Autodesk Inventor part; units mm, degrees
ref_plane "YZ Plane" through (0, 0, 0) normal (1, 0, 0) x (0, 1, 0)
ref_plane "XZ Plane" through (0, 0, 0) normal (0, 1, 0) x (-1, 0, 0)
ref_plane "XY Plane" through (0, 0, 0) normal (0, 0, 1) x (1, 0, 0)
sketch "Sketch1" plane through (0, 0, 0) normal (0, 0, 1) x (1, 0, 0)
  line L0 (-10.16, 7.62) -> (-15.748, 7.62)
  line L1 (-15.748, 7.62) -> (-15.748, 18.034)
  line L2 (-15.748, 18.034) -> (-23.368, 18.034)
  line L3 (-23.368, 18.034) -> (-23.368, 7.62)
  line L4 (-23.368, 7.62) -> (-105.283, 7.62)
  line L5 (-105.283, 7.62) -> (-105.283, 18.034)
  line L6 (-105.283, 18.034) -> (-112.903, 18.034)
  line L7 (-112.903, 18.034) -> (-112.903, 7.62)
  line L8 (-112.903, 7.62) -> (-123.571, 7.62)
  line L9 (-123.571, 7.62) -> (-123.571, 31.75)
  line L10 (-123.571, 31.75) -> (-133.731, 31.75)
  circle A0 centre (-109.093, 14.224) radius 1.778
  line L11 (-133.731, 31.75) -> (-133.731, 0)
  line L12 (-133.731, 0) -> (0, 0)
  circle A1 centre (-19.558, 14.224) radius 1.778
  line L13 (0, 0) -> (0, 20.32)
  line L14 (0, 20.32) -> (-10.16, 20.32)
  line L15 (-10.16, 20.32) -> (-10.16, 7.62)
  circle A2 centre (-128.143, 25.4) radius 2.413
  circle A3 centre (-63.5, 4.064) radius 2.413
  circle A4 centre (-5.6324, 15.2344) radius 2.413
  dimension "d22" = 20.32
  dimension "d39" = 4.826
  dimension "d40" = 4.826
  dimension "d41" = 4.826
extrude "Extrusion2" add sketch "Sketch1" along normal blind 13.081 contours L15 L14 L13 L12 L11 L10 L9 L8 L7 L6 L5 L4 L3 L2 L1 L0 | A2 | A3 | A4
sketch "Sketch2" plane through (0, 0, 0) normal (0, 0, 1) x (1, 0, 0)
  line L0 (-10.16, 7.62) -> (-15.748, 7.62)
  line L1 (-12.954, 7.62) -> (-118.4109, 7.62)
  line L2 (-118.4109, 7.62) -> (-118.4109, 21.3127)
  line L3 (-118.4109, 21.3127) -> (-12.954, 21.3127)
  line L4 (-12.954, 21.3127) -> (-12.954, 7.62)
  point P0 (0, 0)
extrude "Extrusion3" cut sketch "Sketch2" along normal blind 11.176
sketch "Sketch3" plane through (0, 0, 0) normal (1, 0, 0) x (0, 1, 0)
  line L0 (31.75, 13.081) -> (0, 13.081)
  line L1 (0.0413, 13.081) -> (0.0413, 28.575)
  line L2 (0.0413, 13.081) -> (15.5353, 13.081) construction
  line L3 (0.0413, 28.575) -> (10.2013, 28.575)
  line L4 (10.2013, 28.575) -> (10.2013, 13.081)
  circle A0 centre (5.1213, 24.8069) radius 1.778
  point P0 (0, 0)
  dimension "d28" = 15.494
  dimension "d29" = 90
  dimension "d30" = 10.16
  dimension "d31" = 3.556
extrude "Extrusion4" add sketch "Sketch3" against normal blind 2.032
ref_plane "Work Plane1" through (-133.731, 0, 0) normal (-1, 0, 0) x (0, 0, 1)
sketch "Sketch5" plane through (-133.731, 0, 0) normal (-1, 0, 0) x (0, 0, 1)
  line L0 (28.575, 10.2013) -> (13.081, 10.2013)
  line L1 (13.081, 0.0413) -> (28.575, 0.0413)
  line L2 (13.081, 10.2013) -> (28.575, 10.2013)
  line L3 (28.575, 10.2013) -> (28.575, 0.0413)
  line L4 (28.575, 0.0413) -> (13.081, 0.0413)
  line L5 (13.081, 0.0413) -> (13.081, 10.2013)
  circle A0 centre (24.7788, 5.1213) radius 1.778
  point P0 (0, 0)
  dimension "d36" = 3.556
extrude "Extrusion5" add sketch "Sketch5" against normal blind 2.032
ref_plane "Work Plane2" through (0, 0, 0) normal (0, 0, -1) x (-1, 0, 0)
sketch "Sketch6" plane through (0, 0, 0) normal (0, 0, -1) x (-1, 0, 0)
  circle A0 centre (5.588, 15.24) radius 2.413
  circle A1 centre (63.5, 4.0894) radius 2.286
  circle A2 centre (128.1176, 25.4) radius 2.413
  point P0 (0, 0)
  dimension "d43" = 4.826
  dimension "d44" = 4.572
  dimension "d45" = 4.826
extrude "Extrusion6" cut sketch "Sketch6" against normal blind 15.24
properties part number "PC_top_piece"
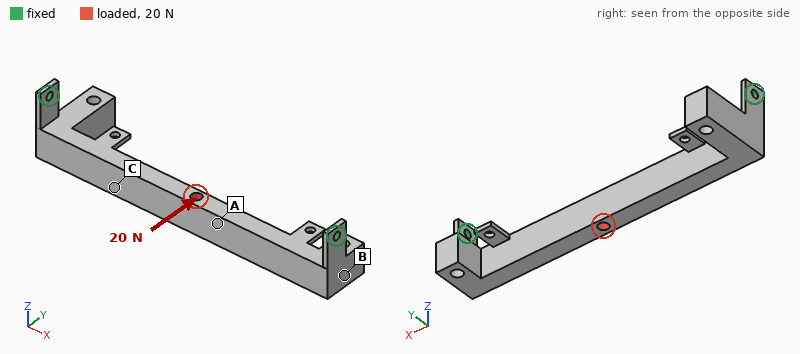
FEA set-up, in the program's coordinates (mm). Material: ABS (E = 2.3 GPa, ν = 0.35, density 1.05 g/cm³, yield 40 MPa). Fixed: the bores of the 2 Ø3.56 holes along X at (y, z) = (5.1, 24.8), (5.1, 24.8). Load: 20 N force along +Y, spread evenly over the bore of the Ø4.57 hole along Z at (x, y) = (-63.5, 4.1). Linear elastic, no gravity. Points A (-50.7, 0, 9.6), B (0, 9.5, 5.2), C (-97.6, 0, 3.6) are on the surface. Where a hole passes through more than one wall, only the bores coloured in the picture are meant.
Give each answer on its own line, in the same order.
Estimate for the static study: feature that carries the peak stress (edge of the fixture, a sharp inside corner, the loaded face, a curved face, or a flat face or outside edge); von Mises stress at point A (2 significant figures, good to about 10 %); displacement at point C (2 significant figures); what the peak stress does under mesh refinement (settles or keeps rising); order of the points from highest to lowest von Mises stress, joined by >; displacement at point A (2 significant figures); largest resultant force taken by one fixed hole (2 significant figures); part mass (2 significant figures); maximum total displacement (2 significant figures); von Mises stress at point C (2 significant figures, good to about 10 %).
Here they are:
edge of the fixture
3.8 MPa
0.66 mm
keeps rising
A > C > B
0.80 mm
11 N
19 g
0.92 mm
2.2 MPa
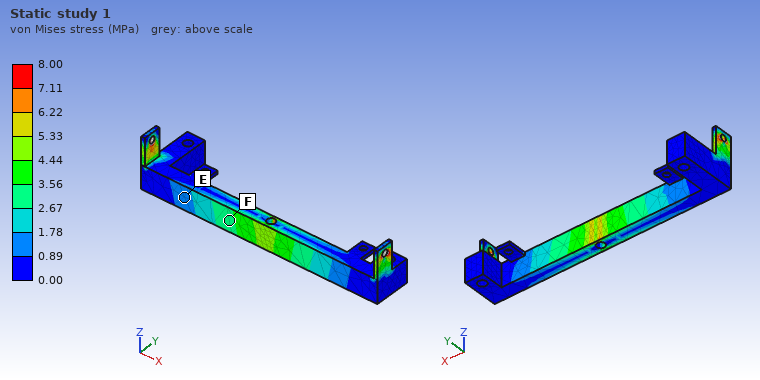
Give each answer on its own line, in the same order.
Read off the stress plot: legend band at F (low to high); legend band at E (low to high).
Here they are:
2.67 to 3.56 MPa
0.89 to 1.78 MPa
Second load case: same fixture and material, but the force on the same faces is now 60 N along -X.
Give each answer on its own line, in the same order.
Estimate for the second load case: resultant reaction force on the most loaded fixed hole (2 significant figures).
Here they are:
31 N
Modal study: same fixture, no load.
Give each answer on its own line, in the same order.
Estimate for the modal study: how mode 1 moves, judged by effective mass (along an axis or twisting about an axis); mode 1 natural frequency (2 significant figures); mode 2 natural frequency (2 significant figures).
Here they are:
along Y
270 Hz
530 Hz
